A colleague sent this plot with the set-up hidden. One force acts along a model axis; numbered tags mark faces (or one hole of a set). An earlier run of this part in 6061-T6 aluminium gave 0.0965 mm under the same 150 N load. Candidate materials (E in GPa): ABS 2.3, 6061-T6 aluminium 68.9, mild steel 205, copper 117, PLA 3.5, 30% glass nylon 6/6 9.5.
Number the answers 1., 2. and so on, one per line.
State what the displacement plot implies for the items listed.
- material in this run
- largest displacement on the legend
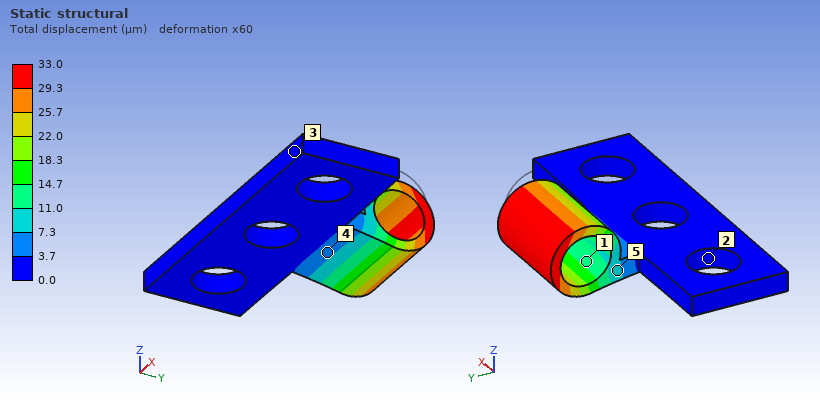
1. mild steel
2. 33.0 µm
